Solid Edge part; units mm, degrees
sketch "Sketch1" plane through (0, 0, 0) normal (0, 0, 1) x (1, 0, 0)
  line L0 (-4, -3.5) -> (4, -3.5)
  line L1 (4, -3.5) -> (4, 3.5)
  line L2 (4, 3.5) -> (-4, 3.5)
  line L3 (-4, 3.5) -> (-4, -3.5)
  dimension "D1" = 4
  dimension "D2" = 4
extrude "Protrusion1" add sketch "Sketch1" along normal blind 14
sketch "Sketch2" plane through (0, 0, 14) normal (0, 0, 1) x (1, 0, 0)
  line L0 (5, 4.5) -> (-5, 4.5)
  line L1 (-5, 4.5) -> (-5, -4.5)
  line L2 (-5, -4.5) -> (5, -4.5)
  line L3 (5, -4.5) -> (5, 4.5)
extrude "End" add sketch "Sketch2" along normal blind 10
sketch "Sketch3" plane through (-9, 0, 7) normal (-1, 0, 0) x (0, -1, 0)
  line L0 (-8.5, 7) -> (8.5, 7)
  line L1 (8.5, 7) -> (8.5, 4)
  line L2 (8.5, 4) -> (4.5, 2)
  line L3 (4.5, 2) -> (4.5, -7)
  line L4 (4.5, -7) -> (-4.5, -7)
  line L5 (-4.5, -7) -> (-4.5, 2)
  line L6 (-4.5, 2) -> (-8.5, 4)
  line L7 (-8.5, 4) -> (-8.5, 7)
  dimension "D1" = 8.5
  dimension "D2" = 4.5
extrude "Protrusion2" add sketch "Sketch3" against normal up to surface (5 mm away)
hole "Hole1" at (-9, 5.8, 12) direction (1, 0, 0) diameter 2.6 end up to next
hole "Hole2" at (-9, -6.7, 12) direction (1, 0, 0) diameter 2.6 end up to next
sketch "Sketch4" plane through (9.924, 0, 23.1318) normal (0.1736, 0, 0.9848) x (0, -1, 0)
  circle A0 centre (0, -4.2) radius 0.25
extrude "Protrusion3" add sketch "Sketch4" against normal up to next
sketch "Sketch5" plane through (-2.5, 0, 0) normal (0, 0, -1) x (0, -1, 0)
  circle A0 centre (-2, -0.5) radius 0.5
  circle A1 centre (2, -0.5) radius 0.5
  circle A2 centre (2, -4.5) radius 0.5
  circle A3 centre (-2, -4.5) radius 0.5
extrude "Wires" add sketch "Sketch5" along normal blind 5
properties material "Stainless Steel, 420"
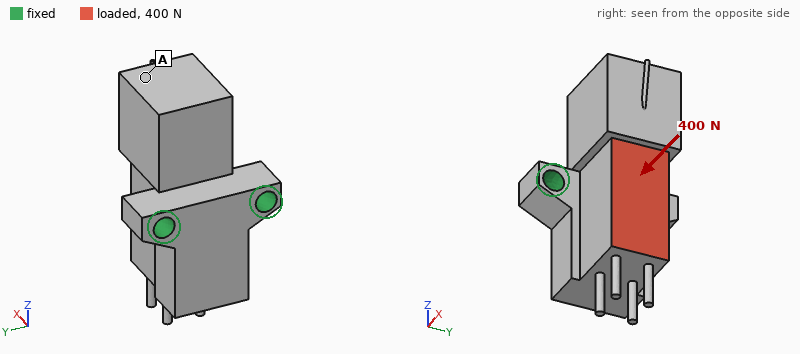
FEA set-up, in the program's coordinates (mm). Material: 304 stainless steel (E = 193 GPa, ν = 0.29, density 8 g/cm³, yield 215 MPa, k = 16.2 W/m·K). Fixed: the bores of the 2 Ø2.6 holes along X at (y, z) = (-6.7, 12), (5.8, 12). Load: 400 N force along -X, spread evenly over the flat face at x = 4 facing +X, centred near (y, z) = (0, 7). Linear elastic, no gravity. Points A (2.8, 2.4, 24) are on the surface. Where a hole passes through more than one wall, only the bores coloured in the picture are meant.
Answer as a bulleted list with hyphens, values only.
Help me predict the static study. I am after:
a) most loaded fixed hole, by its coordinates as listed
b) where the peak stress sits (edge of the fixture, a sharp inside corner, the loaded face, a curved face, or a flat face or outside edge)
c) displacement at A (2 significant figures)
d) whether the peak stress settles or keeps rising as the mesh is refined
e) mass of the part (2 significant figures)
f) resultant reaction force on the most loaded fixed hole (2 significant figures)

- (5.8, 12)
- edge of the fixture
- 5.7 µm
- keeps rising
- 20 g
- 220 N
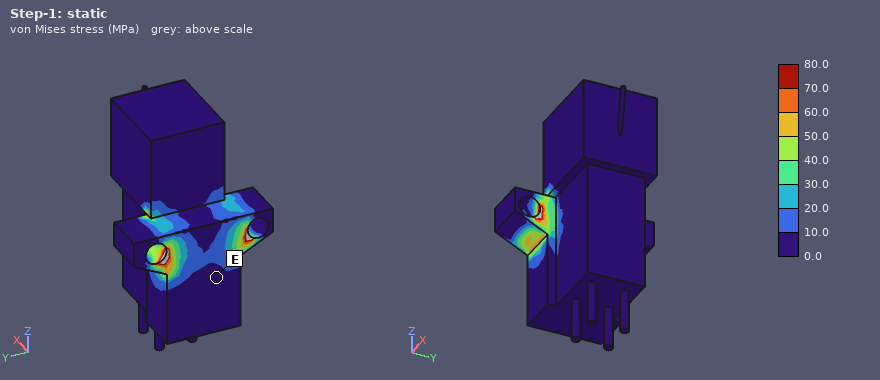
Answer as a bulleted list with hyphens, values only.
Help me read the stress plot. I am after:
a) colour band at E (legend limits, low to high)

- 0.0 to 10.0 MPa
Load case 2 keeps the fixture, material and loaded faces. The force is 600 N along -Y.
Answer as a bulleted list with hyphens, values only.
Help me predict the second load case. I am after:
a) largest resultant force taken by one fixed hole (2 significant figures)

- 720 N
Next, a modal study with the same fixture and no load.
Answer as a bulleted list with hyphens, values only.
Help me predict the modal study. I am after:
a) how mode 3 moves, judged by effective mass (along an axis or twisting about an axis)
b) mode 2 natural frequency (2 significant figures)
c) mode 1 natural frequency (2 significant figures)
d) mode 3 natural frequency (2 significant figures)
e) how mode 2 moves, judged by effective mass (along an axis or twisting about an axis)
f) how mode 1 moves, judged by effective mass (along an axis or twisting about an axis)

- along Y
- 19 kHz
- 8400 Hz
- 22 kHz
- along Y
- along Z
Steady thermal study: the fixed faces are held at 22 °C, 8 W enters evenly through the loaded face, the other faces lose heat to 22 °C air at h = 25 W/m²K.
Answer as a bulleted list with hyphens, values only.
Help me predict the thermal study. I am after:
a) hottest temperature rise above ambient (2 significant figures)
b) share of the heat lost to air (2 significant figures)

- 76 K
- 15 %
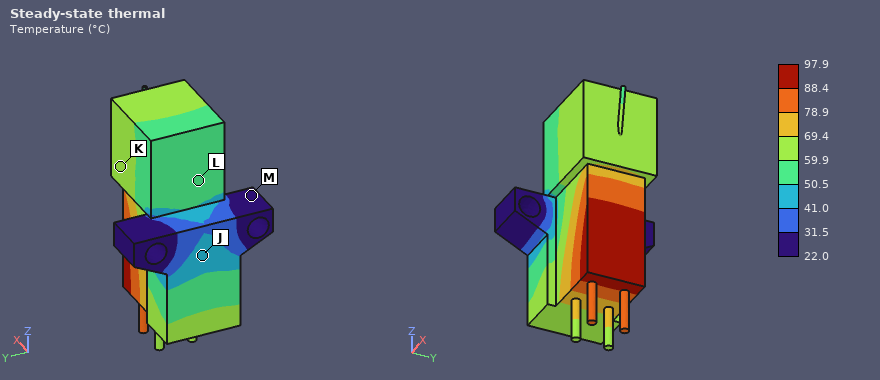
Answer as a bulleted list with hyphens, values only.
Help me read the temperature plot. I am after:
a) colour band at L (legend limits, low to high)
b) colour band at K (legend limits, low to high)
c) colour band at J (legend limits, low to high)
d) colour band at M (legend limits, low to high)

- 50.5 to 59.9 °C
- 59.9 to 69.4 °C
- 41.0 to 50.5 °C
- 22.0 to 31.5 °C
